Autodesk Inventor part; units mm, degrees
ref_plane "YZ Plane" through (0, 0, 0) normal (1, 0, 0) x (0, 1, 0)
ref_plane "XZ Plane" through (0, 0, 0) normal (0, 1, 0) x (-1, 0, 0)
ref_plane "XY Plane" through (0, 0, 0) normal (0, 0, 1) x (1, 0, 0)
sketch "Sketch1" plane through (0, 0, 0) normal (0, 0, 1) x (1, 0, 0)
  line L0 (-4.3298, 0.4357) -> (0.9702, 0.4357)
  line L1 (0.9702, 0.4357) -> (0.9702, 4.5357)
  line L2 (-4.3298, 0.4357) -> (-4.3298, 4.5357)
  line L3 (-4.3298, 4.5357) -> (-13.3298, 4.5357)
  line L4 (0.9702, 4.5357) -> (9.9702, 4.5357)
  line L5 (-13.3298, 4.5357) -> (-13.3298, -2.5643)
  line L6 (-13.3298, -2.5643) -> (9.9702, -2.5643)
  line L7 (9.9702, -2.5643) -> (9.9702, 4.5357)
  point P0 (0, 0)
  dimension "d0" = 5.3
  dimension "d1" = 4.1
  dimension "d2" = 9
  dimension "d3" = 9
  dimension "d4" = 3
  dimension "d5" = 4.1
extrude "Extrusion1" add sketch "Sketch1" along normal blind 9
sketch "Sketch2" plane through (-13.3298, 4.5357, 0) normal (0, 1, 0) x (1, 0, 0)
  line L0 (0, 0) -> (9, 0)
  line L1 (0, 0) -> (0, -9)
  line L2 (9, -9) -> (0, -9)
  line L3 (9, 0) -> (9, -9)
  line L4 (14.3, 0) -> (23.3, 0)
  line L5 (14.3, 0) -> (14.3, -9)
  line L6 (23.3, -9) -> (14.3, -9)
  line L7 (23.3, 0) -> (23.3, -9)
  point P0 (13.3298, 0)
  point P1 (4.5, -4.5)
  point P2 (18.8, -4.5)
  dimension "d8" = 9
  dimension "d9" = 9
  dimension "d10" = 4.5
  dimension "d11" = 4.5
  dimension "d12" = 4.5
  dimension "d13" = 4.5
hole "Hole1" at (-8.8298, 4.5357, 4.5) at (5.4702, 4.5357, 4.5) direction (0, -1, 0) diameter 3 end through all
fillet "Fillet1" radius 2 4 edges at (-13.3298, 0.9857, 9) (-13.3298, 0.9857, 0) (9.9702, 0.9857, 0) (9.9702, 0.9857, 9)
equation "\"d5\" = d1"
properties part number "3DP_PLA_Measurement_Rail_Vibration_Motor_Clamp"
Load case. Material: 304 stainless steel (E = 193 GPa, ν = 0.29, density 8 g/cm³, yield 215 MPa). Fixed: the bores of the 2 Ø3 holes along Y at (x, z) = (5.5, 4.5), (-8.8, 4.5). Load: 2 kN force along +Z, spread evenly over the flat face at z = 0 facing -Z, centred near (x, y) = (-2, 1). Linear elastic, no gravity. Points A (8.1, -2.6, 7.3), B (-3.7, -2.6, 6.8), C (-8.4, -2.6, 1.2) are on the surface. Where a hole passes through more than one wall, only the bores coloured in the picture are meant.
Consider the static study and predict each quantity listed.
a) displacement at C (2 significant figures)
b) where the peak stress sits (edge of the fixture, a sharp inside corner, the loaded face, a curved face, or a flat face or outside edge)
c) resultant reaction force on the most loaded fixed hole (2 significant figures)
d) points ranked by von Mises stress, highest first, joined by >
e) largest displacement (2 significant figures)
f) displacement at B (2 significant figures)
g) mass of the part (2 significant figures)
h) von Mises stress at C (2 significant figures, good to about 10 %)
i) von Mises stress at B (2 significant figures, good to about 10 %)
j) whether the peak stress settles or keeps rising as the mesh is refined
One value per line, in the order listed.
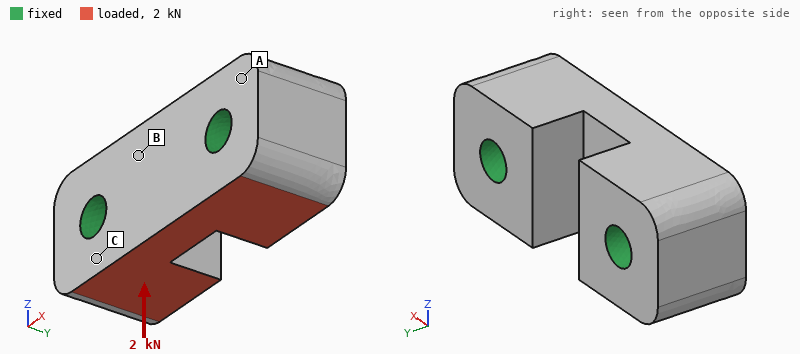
0.30 µm
edge of the fixture
1.0 kN
C > B > A
1.2 µm
0.68 µm
9.3 g
20 MPa
11 MPa
keeps rising
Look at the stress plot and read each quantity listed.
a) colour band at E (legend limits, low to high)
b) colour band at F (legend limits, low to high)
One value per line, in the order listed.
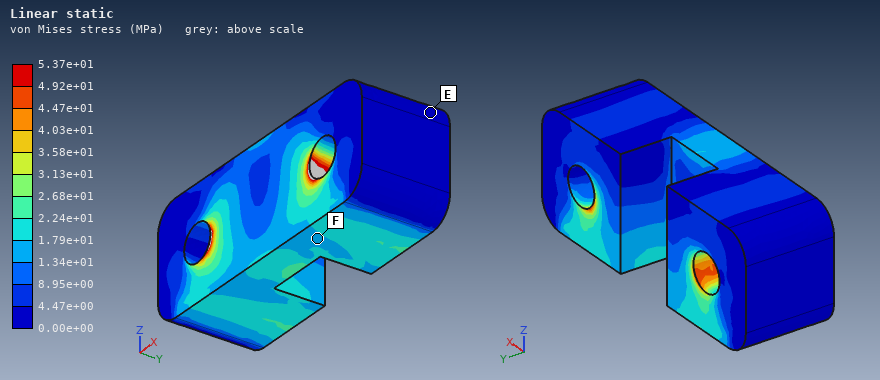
0.00e+00 to 4.47e+00 MPa
1.34e+01 to 1.79e+01 MPa
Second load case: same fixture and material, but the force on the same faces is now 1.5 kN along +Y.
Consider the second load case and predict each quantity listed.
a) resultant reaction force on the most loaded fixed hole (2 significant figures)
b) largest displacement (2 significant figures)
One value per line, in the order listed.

750 N
2.9 µm
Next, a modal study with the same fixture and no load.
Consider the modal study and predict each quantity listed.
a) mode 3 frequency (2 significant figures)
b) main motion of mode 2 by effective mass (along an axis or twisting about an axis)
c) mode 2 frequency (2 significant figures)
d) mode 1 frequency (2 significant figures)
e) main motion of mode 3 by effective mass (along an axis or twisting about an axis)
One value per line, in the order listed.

110 kHz
along Y
100 kHz
89 kHz
twisting about Y
